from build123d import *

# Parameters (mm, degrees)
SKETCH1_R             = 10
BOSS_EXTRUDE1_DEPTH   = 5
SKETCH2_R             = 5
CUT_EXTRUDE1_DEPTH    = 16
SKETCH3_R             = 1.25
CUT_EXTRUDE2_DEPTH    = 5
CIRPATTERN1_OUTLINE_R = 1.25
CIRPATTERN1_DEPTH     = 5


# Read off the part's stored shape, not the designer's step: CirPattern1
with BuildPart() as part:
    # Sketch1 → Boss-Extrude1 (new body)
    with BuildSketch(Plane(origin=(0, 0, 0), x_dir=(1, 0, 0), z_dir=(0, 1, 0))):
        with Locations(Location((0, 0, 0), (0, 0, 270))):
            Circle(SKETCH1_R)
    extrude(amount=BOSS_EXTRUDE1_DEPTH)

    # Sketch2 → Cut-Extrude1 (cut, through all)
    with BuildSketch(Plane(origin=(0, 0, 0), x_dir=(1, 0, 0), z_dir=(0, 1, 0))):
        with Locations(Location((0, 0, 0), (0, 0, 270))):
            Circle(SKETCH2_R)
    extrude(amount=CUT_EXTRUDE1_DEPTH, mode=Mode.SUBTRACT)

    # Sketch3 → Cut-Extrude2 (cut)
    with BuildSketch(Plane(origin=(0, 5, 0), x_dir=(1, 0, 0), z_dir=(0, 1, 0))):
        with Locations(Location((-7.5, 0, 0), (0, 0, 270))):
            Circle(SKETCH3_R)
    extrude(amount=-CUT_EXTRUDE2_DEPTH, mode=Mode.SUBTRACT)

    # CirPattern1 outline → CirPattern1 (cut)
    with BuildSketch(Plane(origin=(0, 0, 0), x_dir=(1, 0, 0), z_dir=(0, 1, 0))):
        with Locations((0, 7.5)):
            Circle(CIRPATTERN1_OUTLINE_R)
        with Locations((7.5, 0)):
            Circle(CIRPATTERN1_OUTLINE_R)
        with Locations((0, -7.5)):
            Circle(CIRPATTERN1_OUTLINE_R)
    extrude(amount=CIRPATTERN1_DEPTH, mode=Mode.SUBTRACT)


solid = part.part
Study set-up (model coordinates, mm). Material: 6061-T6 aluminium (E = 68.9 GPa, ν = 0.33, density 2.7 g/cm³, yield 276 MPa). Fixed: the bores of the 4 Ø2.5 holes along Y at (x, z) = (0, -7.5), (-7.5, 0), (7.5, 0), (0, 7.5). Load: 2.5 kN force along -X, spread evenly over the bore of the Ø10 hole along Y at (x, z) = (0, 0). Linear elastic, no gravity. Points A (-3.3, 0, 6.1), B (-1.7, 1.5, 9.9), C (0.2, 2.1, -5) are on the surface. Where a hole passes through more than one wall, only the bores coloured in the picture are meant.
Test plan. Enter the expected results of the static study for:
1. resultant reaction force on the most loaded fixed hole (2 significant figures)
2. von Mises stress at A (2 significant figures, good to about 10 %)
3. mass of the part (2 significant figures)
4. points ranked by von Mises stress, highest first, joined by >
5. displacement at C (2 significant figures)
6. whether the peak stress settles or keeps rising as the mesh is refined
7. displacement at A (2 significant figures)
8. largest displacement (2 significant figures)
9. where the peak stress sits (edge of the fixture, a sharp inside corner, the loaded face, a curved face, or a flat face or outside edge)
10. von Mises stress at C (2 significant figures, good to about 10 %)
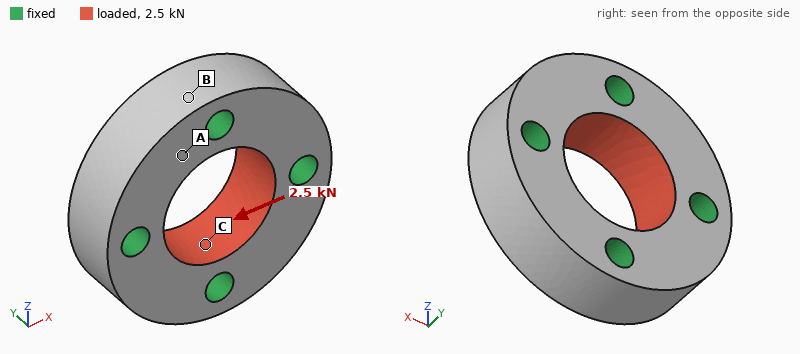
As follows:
660 N
12 MPa
2.9 g
C > A > B
1.3 µm
keeps rising
0.95 µm
1.8 µm
edge of the fixture
28 MPa
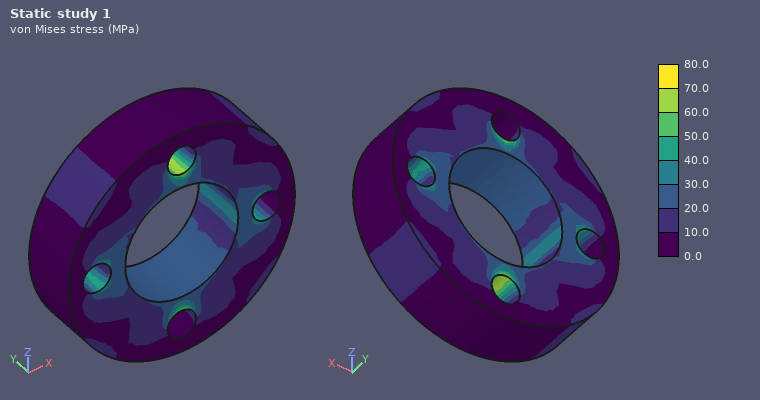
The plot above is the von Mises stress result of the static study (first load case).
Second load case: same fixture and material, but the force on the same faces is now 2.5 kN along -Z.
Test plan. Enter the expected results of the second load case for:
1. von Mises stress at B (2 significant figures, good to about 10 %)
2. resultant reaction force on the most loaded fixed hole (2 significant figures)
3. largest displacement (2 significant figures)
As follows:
6.4 MPa
660 N
1.8 µm
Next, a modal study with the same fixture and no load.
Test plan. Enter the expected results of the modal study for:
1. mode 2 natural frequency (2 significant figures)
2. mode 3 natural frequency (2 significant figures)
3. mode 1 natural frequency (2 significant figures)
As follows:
110 kHz
110 kHz
110 kHz
